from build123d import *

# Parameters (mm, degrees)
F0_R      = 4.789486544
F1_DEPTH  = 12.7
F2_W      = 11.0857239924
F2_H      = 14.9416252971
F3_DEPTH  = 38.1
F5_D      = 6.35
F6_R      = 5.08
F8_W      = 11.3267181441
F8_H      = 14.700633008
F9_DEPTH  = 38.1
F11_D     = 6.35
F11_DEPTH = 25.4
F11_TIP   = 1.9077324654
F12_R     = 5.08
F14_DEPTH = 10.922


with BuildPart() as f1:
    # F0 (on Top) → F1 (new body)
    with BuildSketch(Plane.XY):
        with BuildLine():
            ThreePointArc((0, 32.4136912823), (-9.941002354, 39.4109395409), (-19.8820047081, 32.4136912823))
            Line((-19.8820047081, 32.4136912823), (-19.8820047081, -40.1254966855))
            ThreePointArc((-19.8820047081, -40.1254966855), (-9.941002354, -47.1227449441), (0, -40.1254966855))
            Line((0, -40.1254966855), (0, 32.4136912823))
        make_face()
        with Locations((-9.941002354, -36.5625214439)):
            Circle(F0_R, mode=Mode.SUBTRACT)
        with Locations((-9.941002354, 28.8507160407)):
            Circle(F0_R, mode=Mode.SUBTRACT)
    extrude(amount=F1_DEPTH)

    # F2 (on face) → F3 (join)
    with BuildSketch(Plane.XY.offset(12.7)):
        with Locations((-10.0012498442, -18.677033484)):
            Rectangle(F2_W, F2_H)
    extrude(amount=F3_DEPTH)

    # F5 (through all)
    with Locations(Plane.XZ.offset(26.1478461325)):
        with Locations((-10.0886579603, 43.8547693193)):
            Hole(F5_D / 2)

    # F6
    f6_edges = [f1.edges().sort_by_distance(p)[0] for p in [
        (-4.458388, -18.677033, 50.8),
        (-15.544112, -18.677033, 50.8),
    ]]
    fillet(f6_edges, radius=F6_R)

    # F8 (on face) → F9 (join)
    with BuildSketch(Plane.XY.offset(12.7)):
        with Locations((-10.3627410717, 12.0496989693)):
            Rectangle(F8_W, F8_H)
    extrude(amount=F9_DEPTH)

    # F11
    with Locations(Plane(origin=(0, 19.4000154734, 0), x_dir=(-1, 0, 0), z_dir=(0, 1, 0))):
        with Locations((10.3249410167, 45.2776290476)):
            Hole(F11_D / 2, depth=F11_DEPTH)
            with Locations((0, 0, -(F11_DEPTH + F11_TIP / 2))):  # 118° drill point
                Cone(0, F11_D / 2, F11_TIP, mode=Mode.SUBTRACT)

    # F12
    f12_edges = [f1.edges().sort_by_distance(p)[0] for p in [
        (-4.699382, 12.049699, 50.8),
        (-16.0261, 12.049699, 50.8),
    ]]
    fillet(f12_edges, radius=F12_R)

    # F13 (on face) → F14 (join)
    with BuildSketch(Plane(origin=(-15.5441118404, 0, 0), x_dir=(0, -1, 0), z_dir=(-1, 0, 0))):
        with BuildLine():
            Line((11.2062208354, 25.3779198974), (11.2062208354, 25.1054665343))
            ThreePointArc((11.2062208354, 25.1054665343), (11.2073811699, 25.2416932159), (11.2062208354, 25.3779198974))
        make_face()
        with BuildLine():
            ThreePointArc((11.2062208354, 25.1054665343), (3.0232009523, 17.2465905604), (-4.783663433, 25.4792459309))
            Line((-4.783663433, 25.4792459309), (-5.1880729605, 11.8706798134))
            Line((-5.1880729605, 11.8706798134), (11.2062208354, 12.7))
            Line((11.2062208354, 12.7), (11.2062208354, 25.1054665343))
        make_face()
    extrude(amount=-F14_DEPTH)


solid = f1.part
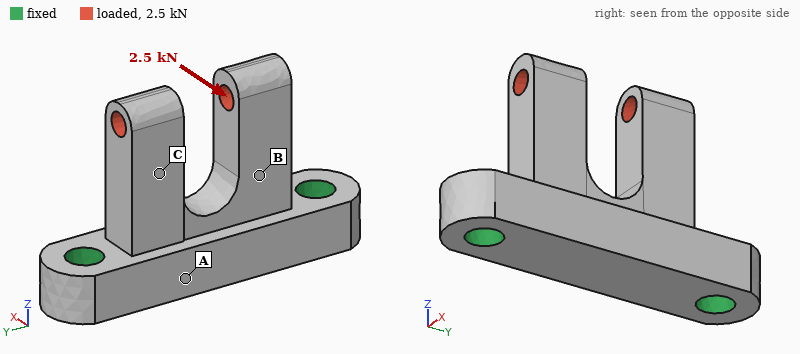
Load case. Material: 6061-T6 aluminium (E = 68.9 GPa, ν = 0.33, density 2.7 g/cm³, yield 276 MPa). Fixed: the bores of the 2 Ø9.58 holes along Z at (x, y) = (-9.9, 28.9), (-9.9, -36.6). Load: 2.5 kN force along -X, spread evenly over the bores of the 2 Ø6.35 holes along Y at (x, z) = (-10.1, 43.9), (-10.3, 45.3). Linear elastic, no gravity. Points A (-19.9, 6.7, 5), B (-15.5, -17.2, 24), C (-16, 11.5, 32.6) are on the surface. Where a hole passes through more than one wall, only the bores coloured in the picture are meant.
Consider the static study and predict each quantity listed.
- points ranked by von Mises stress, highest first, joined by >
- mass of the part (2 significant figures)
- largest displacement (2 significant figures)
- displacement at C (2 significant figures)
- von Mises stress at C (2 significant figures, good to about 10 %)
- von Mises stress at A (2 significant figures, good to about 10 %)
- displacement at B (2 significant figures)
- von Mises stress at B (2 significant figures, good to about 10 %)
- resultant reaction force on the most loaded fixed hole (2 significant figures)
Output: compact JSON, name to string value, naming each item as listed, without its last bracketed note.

{"points ranked by von Mises stress, highest first, joined by >": "B > C > A", "mass of the part": "85 g", "largest displacement": "0.29 mm", "displacement at C": "0.14 mm", "von Mises stress at C": "50 MPa", "von Mises stress at A": "19 MPa", "displacement at B": "0.082 mm", "von Mises stress at B": "76 MPa", "resultant reaction force on the most loaded fixed hole": "1.3 kN"}
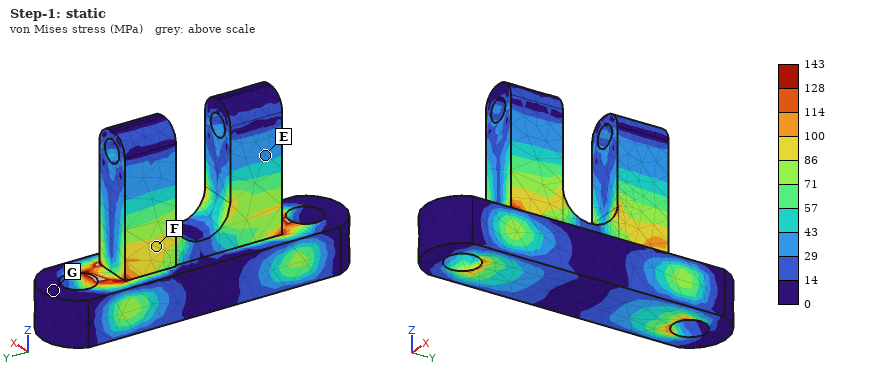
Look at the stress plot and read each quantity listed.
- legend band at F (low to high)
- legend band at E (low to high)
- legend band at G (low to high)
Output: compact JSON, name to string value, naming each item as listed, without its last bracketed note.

{"legend band at F": "86 to 100 MPa", "legend band at E": "29 to 43 MPa", "legend band at G": "0 to 14 MPa"}
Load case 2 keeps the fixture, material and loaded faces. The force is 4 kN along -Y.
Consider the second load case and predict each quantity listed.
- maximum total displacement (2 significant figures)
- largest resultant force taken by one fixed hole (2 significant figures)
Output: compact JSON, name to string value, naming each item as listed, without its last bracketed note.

{"maximum total displacement": "0.15 mm", "largest resultant force taken by one fixed hole": "3.5 kN"}
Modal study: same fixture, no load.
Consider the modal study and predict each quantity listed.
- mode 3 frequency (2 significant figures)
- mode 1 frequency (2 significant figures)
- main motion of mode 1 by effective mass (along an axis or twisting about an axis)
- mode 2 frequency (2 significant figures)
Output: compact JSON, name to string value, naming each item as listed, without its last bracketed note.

{"mode 3 frequency": "7800 Hz", "mode 1 frequency": "4700 Hz", "main motion of mode 1 by effective mass": "along X", "mode 2 frequency": "5900 Hz"}
